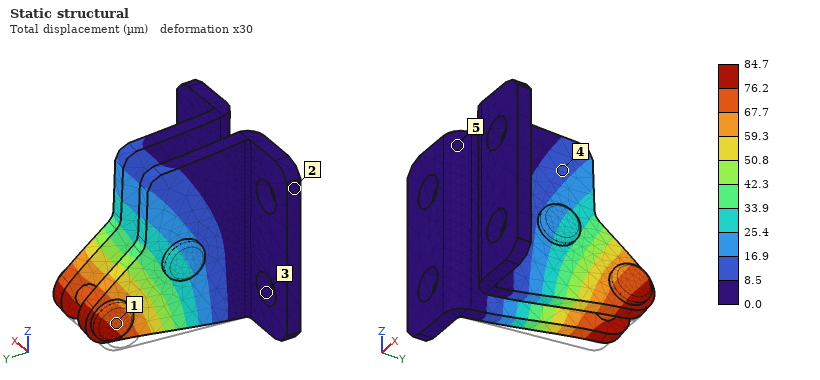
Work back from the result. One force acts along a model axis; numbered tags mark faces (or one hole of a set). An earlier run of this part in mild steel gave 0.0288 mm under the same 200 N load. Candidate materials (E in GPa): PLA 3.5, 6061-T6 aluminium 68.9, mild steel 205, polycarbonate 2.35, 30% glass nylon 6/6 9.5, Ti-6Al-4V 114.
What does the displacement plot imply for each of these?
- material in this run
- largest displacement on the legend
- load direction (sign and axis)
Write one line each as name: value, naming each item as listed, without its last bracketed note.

material in this run: 6061-T6 aluminium
largest displacement on the legend: 84.7 µm
load direction: +X
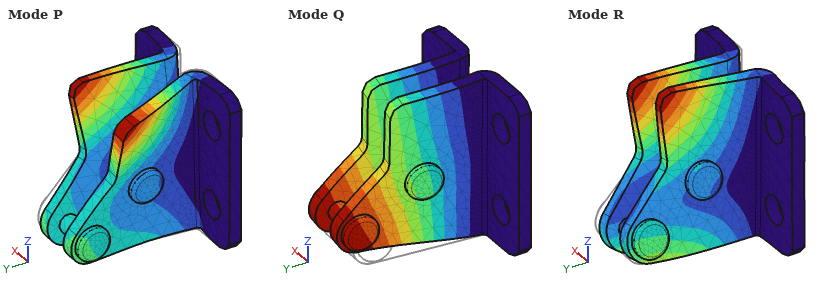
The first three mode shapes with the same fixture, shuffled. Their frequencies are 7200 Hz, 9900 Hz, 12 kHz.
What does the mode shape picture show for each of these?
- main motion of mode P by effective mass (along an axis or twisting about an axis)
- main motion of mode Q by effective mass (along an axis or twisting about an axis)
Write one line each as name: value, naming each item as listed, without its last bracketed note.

main motion of mode P by effective mass: along Z
main motion of mode Q by effective mass: along X
